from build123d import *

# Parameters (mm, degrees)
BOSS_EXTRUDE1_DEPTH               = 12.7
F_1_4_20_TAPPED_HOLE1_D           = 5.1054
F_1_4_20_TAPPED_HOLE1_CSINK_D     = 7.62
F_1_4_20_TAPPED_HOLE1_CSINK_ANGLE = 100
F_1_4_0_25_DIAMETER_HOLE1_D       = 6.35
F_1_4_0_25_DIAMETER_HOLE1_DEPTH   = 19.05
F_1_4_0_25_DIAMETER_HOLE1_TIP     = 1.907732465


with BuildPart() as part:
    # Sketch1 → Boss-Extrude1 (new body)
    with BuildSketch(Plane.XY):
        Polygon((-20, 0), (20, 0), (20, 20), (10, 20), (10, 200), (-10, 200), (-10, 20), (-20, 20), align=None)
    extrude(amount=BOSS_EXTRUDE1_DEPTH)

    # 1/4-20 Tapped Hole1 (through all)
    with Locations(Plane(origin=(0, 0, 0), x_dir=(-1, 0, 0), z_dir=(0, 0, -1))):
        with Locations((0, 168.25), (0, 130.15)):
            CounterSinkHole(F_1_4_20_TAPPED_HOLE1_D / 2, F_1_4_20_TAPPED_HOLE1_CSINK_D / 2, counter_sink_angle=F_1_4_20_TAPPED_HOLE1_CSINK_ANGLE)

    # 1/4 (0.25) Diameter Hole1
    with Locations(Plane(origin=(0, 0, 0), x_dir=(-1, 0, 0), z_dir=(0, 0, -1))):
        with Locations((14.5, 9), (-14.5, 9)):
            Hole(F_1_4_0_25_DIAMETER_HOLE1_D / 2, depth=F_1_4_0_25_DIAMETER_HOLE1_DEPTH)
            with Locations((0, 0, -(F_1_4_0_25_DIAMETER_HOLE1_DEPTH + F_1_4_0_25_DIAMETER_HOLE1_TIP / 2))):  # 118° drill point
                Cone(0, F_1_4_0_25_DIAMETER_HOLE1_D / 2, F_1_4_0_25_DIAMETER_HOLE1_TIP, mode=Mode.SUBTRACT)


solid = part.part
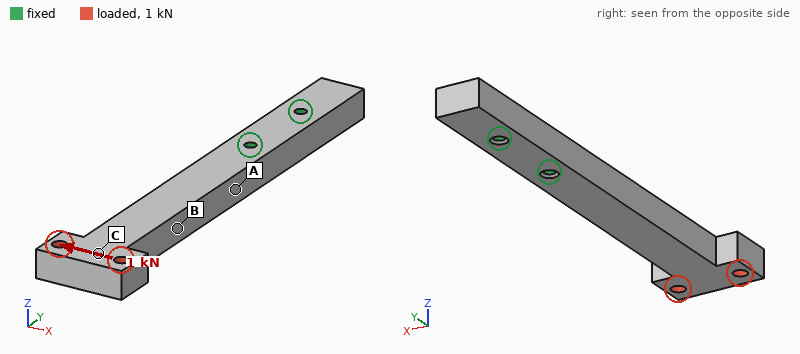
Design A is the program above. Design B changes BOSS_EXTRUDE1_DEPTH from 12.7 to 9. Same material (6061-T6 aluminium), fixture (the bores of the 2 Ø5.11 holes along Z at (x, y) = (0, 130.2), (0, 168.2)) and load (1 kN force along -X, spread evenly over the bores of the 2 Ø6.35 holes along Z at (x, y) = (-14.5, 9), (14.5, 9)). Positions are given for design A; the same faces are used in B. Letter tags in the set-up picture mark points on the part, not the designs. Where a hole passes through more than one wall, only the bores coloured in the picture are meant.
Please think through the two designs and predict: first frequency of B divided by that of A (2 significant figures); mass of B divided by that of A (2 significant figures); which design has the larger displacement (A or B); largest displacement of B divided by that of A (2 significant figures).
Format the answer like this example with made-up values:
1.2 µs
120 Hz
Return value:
0.71
0.71
B
1.4
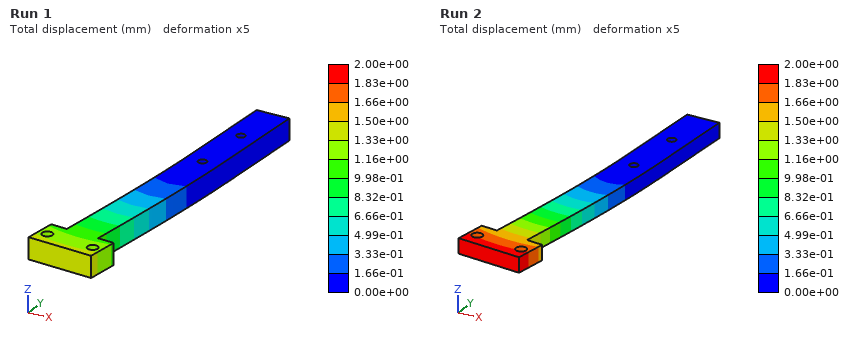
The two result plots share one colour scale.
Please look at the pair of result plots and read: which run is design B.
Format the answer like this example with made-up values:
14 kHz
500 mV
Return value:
Run 2
